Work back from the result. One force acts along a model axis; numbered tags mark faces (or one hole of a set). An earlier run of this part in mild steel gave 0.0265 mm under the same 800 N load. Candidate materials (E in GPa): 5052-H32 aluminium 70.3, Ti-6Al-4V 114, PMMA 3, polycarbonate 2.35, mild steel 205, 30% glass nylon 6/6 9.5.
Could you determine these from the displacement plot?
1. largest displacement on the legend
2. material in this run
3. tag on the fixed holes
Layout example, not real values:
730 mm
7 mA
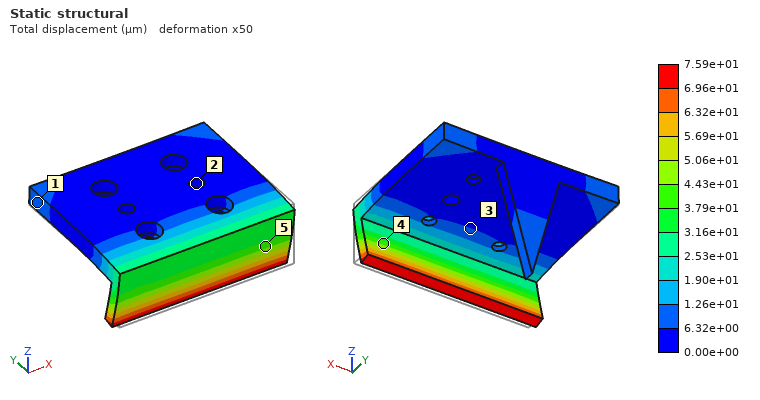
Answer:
7.59e+01 µm
5052-H32 aluminium
2
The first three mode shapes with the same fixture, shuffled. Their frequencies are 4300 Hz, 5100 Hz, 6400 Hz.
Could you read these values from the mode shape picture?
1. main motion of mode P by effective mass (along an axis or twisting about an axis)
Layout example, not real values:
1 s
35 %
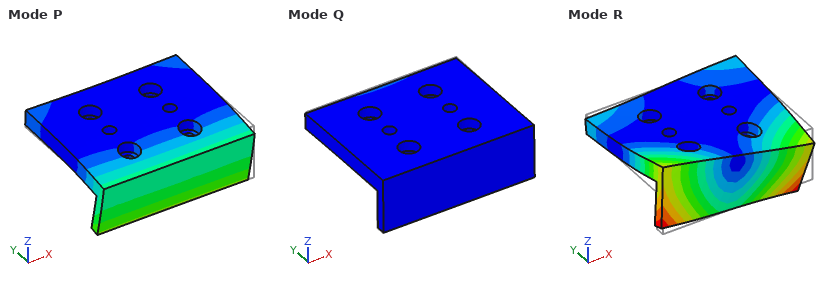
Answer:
along Z
